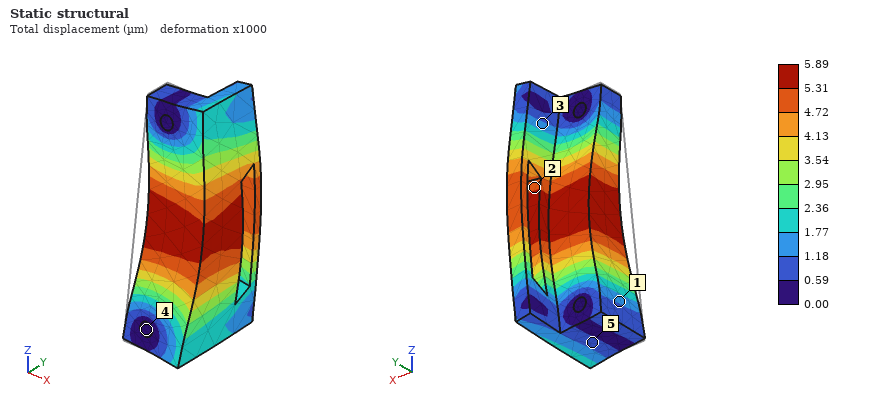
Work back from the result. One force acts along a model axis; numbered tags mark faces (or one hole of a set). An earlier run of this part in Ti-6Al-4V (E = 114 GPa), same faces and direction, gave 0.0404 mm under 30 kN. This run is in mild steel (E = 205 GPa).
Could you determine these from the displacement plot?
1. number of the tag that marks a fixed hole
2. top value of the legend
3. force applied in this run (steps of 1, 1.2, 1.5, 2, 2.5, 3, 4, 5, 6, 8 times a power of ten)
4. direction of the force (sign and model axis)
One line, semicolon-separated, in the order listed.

4; 5.89 µm; 8 kN; +X
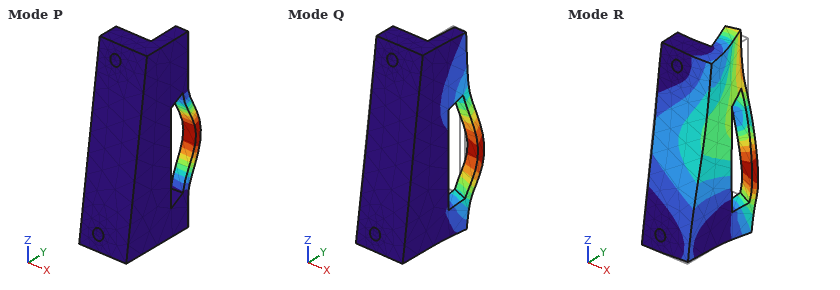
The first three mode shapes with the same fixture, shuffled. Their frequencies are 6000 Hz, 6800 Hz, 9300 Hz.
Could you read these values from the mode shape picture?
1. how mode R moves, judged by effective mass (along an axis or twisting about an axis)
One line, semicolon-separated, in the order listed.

along Y
